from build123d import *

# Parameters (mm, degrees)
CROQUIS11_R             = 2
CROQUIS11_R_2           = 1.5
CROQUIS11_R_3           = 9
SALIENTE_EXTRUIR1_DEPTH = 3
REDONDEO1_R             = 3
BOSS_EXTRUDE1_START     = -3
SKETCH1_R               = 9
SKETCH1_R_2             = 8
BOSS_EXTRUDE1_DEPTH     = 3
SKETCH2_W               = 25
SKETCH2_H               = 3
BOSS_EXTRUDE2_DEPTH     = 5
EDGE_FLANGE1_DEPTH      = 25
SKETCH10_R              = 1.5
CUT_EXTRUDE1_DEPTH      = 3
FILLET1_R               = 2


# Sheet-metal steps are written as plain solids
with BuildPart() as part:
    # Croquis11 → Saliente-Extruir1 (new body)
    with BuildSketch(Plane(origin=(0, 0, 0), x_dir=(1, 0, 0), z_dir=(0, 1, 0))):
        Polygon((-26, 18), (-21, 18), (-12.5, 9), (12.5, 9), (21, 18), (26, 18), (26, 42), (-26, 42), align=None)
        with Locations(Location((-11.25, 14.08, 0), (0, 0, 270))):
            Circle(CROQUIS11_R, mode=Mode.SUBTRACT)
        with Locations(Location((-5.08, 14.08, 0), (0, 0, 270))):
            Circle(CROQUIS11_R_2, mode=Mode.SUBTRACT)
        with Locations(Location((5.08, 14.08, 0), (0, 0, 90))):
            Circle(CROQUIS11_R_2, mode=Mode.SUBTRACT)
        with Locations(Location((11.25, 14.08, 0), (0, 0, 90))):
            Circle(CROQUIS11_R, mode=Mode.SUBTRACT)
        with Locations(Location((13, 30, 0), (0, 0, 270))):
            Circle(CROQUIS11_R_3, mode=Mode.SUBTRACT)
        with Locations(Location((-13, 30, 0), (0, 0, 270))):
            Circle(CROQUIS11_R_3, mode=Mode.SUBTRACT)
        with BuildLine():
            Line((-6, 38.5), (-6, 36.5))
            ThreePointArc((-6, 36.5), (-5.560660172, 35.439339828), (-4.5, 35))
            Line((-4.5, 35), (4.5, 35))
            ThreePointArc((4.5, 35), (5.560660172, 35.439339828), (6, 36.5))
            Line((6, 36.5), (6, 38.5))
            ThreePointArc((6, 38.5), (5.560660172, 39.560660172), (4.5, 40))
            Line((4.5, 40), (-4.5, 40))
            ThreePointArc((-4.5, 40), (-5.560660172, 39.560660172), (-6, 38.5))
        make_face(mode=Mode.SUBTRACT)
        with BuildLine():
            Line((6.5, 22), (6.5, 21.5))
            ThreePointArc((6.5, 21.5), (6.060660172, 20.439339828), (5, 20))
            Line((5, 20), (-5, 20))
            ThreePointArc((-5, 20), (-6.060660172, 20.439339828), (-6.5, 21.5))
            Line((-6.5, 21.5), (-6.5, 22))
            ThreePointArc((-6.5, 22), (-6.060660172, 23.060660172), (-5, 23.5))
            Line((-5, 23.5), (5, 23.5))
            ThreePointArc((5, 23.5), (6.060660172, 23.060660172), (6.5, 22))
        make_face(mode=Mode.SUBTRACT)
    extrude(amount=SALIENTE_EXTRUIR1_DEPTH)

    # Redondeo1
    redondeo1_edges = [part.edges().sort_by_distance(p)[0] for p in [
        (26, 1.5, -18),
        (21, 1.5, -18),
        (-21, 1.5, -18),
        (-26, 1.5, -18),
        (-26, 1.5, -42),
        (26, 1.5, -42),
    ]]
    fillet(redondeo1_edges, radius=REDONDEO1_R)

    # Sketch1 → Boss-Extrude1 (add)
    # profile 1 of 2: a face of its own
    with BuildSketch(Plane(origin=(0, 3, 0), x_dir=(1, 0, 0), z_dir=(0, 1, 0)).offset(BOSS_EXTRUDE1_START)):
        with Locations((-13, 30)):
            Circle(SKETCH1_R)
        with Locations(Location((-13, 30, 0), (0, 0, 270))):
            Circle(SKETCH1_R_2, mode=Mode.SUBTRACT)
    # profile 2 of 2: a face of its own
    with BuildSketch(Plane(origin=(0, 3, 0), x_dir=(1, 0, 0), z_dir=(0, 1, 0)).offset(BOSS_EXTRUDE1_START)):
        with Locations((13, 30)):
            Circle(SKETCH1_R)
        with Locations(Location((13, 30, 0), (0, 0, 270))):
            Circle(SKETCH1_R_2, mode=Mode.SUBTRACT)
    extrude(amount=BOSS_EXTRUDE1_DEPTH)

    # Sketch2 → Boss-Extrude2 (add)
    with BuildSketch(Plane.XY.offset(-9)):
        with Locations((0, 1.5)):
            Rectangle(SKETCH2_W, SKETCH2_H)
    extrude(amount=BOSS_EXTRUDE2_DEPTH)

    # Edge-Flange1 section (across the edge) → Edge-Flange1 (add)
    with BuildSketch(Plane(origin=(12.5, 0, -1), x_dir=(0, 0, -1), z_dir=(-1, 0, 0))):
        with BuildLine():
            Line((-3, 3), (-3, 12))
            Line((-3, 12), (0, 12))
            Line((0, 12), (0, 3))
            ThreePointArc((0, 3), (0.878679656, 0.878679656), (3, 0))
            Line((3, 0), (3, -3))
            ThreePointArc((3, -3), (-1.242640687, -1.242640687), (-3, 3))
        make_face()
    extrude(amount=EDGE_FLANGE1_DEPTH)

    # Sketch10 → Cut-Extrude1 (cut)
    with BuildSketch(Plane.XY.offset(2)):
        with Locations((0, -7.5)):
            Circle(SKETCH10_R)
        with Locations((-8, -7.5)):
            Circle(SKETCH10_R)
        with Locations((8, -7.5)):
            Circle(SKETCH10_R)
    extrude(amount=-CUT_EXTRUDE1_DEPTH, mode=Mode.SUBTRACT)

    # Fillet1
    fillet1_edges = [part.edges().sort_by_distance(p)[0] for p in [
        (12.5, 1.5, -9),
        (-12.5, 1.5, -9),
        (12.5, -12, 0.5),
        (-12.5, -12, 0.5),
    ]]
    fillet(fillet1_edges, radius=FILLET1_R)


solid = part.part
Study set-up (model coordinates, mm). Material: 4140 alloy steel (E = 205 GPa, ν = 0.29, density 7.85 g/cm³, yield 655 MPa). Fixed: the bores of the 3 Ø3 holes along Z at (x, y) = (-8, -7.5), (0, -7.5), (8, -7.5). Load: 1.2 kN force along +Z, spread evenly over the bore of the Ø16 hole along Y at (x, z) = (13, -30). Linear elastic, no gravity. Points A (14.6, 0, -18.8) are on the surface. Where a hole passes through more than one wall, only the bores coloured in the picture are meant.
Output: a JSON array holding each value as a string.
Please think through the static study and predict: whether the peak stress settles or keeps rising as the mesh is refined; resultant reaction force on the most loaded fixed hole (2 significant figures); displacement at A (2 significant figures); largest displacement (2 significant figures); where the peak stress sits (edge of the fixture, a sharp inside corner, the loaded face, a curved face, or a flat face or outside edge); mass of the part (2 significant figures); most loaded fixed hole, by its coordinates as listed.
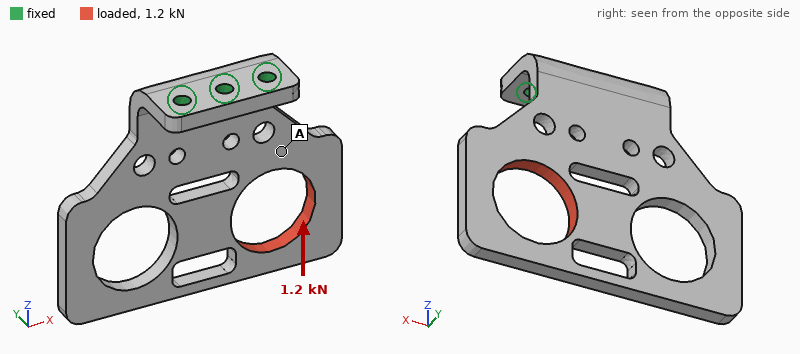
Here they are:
["keeps rising", "1.2 kN", "0.13 mm", "0.26 mm", "edge of the fixture", "35 g", "(8, -7.5)"]
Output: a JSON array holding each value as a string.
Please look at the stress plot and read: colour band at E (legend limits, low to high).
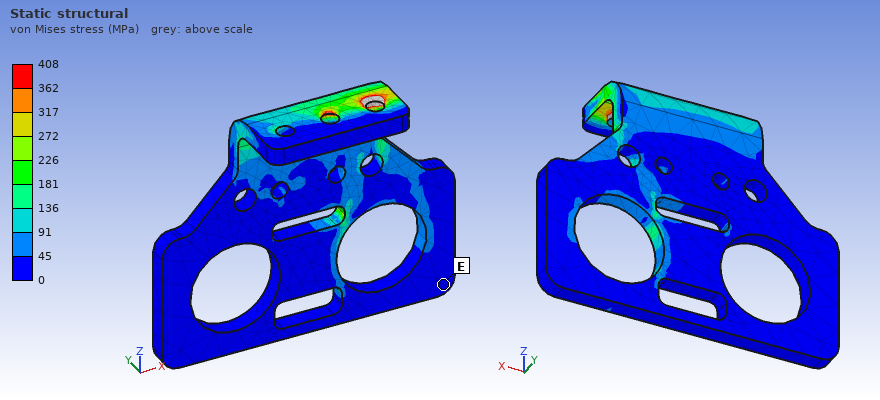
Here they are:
["0 to 45 MPa"]
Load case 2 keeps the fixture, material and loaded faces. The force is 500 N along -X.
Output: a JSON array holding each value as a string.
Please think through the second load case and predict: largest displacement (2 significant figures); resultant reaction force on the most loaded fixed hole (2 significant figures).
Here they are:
["0.14 mm", "860 N"]
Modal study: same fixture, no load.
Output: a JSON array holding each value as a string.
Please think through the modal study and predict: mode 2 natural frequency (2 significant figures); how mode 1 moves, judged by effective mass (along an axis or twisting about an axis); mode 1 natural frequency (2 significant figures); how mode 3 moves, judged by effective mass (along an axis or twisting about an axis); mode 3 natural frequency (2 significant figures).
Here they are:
["1700 Hz", "along Y", "940 Hz", "along X", "2700 Hz"]
